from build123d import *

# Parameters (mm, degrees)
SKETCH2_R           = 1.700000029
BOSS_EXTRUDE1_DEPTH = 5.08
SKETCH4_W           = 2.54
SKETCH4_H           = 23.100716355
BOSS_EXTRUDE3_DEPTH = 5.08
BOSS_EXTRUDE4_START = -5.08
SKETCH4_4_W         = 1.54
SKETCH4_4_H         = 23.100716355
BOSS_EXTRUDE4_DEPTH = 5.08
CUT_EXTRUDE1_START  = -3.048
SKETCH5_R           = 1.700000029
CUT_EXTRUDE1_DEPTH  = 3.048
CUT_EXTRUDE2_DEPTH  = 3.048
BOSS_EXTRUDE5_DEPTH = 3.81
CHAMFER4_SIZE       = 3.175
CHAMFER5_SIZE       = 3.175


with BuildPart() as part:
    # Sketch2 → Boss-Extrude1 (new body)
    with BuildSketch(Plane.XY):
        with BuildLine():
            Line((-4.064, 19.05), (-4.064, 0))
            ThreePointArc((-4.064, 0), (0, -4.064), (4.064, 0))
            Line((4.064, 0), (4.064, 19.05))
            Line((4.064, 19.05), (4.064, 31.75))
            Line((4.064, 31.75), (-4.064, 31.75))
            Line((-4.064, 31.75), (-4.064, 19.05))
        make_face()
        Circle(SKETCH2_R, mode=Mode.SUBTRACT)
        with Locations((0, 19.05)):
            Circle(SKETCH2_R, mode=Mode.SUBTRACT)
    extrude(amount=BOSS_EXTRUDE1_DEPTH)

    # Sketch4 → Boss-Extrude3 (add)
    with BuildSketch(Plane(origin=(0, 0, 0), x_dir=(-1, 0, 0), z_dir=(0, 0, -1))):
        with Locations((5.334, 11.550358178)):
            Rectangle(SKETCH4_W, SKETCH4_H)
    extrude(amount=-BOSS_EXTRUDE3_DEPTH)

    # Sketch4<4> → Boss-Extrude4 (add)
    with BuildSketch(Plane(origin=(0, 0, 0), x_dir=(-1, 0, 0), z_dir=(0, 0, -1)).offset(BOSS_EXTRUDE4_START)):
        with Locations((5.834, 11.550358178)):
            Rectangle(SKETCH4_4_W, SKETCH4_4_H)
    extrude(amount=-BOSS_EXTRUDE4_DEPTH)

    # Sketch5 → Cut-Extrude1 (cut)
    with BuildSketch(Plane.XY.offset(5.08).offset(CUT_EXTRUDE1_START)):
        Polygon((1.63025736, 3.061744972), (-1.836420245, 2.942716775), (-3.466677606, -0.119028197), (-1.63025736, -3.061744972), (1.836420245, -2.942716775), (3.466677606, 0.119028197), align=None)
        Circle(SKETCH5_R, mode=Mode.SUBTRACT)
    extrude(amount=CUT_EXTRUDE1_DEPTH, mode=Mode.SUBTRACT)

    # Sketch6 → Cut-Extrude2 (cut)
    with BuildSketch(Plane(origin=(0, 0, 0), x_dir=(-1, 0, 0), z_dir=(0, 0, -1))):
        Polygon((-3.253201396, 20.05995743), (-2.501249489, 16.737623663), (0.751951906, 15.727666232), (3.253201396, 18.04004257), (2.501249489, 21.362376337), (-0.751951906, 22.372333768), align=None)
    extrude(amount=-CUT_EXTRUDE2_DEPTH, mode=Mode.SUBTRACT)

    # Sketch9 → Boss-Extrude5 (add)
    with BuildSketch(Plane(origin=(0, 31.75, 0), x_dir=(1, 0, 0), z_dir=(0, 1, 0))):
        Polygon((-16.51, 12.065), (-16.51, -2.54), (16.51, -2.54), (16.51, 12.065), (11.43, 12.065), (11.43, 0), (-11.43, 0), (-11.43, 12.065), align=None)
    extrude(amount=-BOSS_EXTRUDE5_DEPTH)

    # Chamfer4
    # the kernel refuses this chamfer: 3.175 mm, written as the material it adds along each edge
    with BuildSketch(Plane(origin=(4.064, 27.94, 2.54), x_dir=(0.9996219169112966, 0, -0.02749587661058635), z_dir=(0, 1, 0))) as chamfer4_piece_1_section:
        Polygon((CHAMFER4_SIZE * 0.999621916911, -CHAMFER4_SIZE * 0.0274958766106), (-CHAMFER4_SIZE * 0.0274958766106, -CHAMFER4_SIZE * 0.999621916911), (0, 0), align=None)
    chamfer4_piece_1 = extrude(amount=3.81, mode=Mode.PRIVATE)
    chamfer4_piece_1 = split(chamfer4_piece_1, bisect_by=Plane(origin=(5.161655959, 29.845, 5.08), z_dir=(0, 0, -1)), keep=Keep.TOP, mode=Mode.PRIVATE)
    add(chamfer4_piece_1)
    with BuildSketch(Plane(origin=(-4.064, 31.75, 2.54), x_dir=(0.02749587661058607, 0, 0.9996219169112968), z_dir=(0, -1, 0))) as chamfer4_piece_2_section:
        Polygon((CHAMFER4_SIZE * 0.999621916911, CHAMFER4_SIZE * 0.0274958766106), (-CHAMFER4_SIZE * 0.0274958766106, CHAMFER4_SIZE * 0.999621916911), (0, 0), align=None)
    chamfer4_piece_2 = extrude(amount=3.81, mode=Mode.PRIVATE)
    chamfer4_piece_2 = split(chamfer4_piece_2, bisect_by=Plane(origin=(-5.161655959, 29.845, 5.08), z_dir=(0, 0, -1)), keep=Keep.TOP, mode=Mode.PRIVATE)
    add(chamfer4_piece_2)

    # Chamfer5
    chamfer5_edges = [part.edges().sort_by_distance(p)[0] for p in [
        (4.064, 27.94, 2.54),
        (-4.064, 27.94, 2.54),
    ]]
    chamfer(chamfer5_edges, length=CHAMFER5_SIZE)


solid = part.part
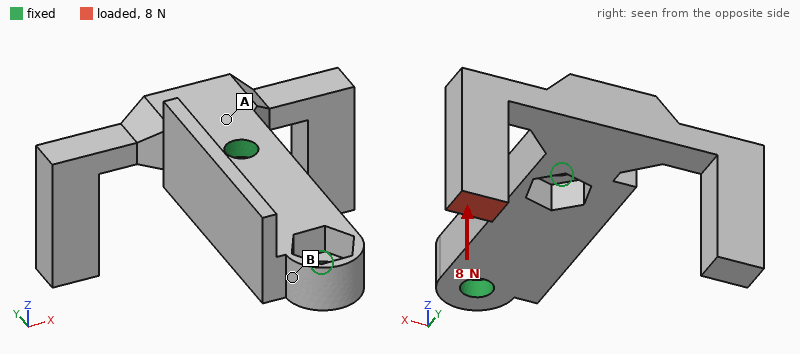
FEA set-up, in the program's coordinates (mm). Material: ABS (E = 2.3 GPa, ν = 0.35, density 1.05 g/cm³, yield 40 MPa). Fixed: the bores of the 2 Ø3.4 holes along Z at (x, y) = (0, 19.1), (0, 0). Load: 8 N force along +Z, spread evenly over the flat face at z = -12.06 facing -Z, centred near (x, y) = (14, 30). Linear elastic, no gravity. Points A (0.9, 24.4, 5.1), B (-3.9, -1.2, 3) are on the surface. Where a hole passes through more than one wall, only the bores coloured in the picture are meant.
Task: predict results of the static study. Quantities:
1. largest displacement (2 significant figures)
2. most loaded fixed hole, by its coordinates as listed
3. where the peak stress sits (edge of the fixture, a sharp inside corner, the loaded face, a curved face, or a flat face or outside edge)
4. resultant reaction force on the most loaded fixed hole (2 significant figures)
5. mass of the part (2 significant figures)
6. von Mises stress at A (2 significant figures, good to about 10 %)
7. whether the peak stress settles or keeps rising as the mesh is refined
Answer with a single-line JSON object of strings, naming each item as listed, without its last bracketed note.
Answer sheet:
{"largest displacement": "0.56 mm", "most loaded fixed hole, by its coordinates as listed": "(0, 19.1)", "where the peak stress sits": "edge of the fixture", "resultant reaction force on the most loaded fixed hole": "10 N", "mass of the part": "2.6 g", "von Mises stress at A": "4.3 MPa", "whether the peak stress settles or keeps rising as the mesh is refined": "keeps rising"}
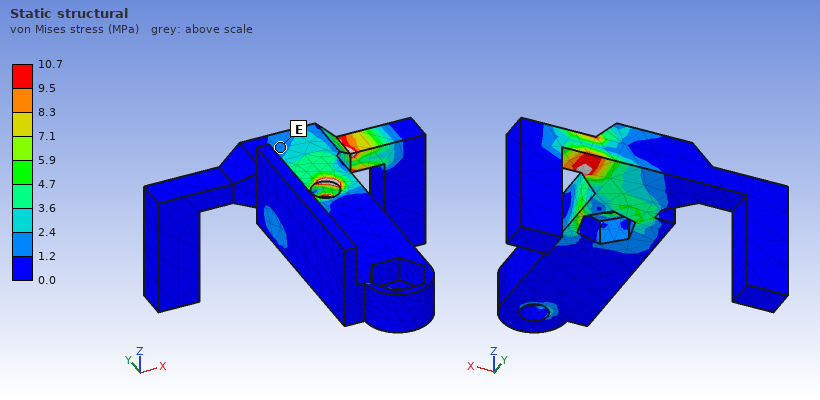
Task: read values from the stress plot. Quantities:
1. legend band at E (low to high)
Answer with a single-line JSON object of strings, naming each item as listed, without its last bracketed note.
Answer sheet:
{"legend band at E": "1.2 to 2.4 MPa"}
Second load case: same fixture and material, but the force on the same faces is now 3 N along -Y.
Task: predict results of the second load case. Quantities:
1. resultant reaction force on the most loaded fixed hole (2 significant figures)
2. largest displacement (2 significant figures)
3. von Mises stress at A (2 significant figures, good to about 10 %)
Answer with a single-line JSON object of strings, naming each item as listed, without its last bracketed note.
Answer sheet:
{"resultant reaction force on the most loaded fixed hole": "2.6 N", "largest displacement": "0.44 mm", "von Mises stress at A": "1.1 MPa"}
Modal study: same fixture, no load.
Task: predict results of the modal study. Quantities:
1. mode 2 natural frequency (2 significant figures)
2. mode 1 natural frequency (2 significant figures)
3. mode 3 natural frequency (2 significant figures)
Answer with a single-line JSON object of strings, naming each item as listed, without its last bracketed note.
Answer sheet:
{"mode 2 natural frequency": "1200 Hz", "mode 1 natural frequency": "1000 Hz", "mode 3 natural frequency": "1300 Hz"}
